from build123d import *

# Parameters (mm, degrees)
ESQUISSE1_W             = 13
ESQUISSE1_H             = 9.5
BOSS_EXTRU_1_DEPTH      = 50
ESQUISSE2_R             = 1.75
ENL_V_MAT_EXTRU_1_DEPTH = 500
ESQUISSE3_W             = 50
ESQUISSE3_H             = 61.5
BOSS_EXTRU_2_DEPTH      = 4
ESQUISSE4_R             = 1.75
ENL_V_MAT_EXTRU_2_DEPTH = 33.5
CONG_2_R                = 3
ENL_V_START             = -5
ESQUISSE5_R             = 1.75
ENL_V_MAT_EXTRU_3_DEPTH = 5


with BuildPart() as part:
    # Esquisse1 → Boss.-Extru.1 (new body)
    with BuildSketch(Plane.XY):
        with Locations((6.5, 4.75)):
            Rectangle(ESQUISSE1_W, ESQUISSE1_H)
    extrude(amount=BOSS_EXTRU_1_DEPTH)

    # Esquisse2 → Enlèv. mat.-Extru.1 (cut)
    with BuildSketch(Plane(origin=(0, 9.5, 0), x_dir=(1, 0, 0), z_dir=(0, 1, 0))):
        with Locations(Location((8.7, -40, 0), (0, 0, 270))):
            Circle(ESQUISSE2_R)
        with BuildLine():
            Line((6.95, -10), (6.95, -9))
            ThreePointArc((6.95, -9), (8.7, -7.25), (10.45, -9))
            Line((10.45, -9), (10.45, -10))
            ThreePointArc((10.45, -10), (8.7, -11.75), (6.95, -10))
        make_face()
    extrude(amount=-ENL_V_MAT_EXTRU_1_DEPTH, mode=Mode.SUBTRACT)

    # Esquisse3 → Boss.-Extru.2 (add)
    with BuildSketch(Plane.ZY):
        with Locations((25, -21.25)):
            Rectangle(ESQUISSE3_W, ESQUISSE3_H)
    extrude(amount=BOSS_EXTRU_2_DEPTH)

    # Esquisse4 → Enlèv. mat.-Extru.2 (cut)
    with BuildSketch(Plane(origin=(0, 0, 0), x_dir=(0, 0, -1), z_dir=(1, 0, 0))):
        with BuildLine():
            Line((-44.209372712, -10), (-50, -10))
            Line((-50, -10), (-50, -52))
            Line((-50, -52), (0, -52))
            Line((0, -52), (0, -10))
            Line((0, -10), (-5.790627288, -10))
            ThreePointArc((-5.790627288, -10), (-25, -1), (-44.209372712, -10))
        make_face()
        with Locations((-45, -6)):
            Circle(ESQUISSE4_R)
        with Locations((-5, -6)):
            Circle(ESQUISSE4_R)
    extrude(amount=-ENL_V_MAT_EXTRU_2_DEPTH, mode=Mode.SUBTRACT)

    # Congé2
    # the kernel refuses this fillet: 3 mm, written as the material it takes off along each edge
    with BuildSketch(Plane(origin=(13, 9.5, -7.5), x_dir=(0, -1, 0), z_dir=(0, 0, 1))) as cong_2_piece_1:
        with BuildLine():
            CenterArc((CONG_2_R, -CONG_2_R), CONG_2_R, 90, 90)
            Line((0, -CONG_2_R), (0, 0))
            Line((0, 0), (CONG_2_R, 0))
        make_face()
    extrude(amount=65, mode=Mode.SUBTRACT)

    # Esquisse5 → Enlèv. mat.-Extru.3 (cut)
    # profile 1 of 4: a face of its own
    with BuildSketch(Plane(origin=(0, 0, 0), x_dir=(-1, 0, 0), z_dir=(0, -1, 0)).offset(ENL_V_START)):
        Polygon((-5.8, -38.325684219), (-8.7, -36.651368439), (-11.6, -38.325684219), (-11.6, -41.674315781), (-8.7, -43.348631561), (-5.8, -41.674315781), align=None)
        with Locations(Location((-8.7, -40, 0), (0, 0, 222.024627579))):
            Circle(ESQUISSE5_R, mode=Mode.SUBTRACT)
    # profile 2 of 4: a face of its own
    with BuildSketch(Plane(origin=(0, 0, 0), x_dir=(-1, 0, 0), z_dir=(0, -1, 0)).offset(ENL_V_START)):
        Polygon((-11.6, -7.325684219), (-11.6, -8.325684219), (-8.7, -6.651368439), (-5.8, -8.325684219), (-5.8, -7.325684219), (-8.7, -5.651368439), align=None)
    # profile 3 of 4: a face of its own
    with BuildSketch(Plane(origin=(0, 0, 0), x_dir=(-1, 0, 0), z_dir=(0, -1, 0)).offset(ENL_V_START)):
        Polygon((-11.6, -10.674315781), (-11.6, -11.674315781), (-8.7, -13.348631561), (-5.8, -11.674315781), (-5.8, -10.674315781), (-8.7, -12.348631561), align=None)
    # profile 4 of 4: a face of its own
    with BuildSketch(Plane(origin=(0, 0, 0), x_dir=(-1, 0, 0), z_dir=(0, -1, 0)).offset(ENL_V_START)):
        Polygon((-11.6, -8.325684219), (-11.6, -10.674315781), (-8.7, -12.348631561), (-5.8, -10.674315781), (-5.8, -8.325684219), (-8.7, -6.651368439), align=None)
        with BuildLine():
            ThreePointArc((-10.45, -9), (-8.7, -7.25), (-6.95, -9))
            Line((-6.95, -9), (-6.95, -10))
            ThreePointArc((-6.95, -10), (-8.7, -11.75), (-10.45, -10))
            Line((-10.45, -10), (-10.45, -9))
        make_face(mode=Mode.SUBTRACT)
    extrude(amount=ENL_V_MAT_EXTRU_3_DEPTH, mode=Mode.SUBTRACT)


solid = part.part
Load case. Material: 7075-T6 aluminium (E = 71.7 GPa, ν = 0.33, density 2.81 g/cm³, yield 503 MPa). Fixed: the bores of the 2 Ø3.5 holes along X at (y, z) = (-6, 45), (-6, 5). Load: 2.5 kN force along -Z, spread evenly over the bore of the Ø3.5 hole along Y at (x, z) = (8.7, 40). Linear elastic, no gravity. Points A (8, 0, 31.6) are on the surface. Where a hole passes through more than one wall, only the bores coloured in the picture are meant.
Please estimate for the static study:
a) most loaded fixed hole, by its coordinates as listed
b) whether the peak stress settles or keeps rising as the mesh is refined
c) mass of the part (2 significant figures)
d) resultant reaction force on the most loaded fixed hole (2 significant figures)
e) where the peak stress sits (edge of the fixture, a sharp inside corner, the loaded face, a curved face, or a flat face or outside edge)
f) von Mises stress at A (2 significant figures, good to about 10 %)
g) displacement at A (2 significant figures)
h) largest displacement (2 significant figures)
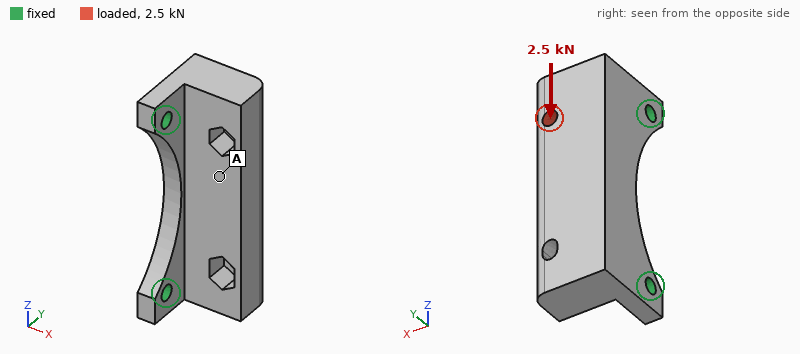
(-6, 5)
keeps rising
24 g
1.7 kN
edge of the fixture
13 MPa
20 µm
34 µm
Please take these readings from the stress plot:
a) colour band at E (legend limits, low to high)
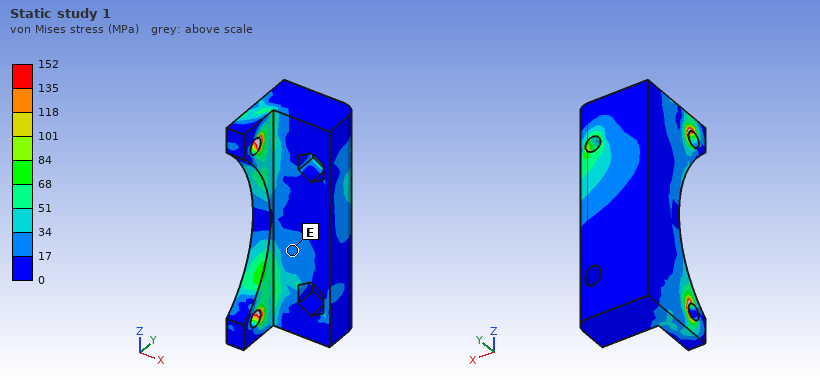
17 to 34 MPa
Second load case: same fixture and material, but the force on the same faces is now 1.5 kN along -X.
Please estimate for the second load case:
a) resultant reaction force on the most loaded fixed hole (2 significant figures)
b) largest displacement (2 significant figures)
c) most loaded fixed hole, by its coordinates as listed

1.3 kN
0.23 mm
(-6, 45)
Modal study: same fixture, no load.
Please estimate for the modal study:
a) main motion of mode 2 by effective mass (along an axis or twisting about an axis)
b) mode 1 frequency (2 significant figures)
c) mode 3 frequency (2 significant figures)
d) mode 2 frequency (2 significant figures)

along Z
3500 Hz
14 kHz
11 kHz
